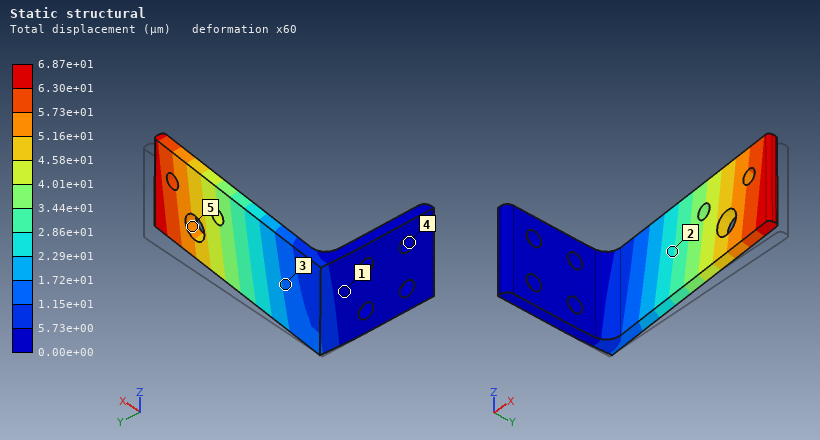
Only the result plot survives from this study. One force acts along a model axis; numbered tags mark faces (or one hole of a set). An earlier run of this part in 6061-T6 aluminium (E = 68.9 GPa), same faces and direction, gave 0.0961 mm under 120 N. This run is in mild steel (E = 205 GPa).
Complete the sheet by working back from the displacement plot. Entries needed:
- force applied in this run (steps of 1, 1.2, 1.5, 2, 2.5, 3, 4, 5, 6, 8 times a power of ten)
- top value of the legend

250 N
6.87e+01 µm
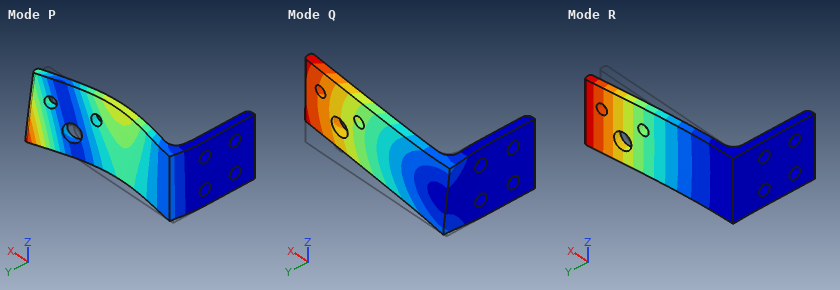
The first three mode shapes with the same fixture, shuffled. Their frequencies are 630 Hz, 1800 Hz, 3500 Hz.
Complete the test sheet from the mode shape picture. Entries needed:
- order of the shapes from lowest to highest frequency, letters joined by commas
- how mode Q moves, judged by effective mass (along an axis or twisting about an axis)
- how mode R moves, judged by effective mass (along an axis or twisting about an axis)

R, Q, P
along Z
along Y
